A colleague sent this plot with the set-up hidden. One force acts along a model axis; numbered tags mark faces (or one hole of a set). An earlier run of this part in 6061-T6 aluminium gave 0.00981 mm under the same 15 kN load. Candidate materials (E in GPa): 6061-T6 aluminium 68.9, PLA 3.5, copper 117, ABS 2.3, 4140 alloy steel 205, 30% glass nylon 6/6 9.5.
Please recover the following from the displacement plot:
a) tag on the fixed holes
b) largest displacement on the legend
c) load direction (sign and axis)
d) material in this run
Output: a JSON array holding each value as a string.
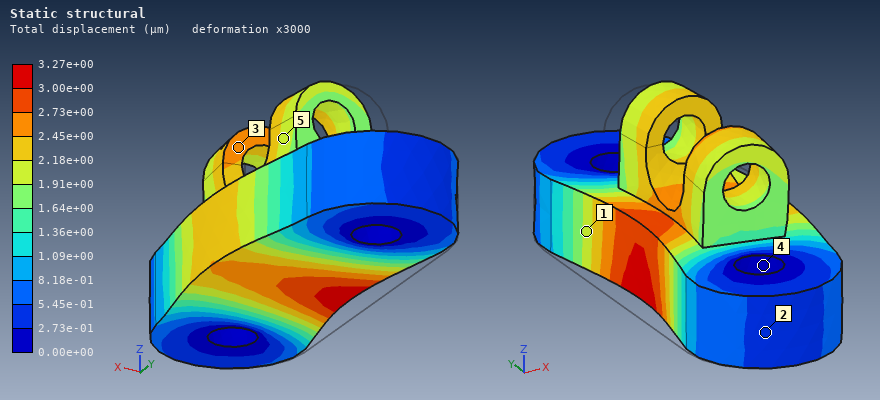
["4", "3.27e+00 µm", "+X", "4140 alloy steel"]
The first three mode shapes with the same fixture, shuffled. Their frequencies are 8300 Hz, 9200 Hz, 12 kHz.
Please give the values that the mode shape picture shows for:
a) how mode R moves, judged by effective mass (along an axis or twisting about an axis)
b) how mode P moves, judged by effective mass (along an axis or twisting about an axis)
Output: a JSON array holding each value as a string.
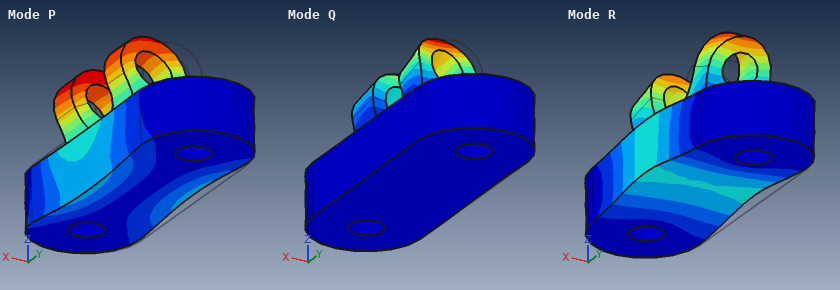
["along Z", "along X"]
